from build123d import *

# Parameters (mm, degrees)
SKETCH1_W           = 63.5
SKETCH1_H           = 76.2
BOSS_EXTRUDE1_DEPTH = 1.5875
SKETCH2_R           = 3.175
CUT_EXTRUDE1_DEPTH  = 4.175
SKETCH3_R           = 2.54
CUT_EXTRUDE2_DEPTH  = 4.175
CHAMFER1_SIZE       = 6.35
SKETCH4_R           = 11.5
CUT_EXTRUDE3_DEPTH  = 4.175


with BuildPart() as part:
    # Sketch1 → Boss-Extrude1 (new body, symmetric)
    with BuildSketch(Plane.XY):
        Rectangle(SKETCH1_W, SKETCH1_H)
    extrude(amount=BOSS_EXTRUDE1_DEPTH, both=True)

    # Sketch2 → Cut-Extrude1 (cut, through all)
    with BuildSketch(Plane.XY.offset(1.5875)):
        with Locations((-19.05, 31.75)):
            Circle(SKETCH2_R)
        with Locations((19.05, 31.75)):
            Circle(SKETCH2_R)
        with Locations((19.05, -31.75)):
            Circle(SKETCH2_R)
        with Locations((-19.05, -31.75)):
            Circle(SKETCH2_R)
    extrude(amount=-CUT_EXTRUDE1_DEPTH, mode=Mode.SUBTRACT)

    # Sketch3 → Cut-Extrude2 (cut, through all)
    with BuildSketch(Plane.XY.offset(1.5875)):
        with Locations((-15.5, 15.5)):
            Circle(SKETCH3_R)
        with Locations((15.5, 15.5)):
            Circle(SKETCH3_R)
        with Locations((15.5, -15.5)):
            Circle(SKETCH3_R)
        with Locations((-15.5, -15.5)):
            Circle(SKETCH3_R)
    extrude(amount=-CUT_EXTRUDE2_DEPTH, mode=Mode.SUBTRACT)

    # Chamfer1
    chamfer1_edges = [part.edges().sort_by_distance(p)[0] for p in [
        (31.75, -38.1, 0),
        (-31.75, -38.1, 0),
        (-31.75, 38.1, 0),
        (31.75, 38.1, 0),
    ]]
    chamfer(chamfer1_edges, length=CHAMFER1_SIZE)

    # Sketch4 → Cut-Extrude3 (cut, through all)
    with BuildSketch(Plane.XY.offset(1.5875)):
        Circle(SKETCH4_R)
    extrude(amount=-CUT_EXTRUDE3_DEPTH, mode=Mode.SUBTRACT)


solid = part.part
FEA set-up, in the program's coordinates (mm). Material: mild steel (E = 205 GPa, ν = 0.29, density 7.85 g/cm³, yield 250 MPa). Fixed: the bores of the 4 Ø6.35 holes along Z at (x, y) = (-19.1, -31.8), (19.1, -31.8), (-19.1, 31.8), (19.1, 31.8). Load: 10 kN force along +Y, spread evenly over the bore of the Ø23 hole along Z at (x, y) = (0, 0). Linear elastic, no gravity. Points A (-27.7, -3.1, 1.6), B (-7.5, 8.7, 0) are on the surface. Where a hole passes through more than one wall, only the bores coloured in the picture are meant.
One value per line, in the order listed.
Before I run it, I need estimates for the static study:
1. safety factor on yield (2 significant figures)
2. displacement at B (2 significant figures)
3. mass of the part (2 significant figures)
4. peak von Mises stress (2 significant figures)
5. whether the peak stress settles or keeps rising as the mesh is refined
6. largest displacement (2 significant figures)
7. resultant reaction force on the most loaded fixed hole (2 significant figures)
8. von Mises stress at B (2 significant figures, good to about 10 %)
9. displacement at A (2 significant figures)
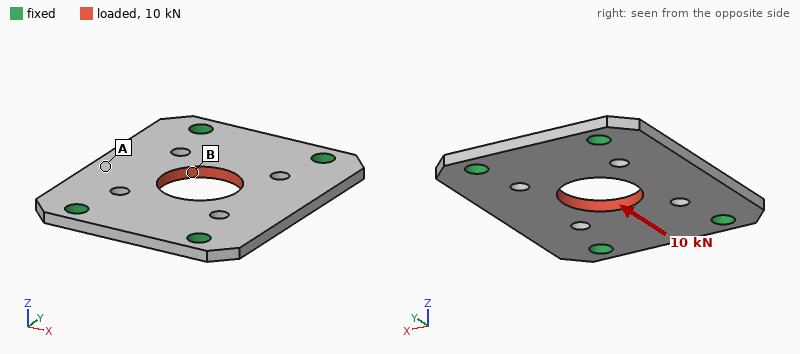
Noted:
2.0
6.5 µm
100 g
120 MPa
settles
7.0 µm
2.6 kN
58 MPa
2.4 µm
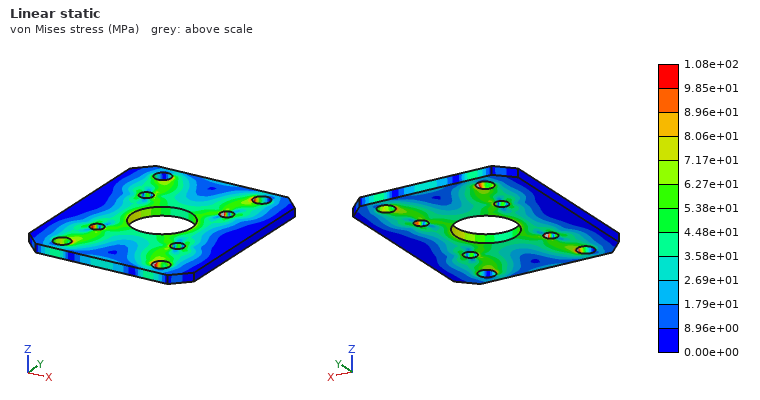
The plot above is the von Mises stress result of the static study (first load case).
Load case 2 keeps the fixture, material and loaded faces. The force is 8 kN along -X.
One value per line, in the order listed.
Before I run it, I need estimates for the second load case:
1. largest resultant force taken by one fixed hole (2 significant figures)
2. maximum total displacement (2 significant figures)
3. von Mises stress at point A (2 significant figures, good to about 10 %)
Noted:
2.2 kN
11 µm
31 MPa
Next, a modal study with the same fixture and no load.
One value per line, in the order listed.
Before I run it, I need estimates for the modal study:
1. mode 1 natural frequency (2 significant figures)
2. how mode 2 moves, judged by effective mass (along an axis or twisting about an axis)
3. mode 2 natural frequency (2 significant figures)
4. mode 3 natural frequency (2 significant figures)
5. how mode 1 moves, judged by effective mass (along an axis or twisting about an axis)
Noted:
4400 Hz
twisting about Y
4900 Hz
7100 Hz
along Z
